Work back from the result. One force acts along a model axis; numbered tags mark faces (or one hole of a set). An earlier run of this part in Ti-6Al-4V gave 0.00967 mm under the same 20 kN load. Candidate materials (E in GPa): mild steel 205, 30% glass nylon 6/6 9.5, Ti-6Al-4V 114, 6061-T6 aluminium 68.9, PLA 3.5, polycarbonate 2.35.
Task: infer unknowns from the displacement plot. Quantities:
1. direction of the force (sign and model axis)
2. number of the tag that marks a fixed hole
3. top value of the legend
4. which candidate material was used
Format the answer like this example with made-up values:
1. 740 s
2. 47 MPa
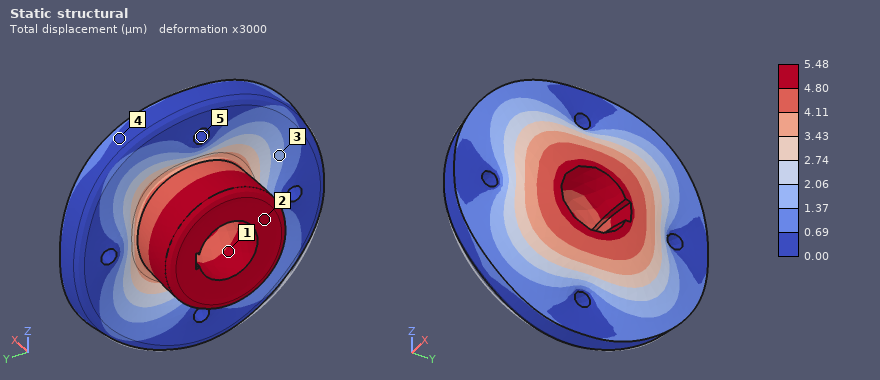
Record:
1. +X
2. 5
3. 5.48 µm
4. mild steel
